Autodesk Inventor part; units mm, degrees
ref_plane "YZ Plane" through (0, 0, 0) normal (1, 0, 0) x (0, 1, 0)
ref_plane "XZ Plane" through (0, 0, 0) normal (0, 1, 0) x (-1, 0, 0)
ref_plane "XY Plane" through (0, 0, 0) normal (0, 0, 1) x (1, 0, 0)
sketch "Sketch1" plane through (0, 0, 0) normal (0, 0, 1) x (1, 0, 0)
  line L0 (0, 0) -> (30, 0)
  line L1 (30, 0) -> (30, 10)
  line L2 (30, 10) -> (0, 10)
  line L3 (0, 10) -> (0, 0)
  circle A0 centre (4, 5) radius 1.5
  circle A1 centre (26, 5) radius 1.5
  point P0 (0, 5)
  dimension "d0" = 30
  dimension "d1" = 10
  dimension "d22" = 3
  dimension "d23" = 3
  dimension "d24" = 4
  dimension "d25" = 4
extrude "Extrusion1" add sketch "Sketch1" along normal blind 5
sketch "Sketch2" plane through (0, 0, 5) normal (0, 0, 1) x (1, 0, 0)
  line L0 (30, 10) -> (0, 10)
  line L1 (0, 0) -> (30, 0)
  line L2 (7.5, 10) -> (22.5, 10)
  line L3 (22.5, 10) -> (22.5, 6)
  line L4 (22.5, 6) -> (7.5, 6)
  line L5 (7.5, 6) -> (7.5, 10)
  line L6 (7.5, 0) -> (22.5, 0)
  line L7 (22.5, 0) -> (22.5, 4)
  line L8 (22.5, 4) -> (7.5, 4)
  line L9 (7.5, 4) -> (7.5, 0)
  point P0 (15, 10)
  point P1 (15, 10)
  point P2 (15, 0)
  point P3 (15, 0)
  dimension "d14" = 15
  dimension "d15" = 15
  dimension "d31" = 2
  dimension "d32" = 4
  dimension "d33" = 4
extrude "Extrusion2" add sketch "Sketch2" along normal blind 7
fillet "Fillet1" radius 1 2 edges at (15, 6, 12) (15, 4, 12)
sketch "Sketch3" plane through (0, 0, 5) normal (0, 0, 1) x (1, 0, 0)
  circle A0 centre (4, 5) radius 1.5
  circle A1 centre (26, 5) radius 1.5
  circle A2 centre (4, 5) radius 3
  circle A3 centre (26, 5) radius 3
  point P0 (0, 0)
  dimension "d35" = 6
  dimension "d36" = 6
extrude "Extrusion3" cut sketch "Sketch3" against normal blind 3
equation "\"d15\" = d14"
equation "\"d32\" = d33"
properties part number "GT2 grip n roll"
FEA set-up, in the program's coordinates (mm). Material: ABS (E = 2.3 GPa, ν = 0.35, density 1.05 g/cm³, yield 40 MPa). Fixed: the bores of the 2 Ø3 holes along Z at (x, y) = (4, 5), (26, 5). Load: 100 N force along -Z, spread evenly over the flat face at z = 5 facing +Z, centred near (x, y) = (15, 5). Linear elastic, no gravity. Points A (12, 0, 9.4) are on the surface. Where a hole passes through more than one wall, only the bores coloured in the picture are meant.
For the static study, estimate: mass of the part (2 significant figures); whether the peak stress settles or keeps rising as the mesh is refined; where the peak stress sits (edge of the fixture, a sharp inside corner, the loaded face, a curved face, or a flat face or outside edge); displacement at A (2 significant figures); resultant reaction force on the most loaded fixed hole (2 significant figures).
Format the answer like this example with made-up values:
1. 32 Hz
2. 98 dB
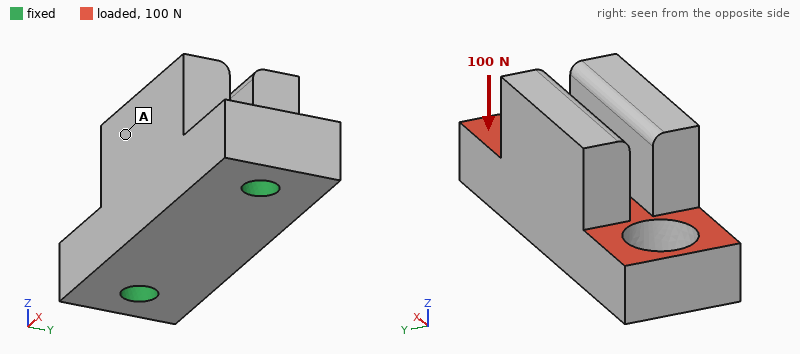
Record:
1. 2.2 g
2. keeps rising
3. edge of the fixture
4. 9.9 µm
5. 50 N
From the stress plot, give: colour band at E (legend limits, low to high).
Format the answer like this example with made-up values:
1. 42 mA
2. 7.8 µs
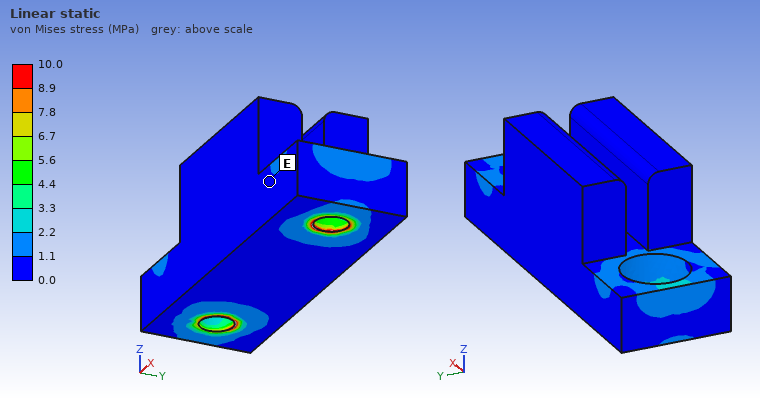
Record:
1. 0.0 to 1.1 MPa
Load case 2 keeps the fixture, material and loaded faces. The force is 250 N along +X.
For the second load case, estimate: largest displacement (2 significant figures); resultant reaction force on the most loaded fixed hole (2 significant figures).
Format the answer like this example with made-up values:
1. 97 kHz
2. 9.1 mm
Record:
1. 59 µm
2. 130 N
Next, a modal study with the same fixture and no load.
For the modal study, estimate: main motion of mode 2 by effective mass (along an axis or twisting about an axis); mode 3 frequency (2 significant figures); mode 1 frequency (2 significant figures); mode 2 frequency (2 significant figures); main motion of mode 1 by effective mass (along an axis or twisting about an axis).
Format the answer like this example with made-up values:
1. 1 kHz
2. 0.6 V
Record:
1. along Z
2. 10 kHz
3. 3300 Hz
4. 8300 Hz
5. along Y
